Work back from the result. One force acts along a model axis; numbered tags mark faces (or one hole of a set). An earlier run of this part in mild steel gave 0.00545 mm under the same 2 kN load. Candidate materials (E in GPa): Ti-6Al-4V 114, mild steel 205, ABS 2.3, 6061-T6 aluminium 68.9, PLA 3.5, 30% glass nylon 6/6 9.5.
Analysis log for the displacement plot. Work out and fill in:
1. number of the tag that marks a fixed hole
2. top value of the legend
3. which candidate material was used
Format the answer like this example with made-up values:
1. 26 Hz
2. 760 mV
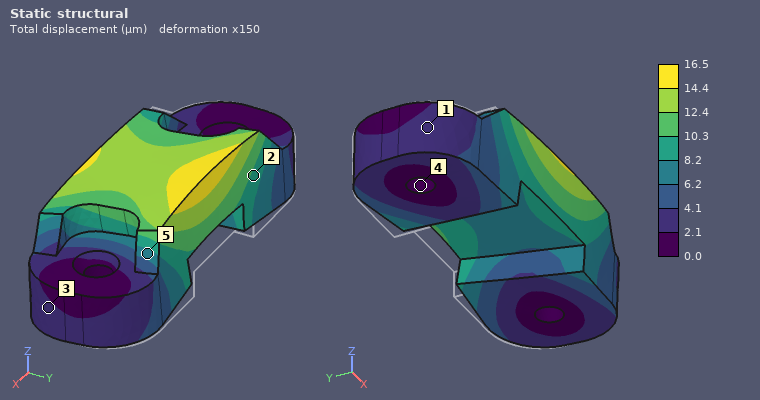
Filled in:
1. 4
2. 16.5 µm
3. 6061-T6 aluminium
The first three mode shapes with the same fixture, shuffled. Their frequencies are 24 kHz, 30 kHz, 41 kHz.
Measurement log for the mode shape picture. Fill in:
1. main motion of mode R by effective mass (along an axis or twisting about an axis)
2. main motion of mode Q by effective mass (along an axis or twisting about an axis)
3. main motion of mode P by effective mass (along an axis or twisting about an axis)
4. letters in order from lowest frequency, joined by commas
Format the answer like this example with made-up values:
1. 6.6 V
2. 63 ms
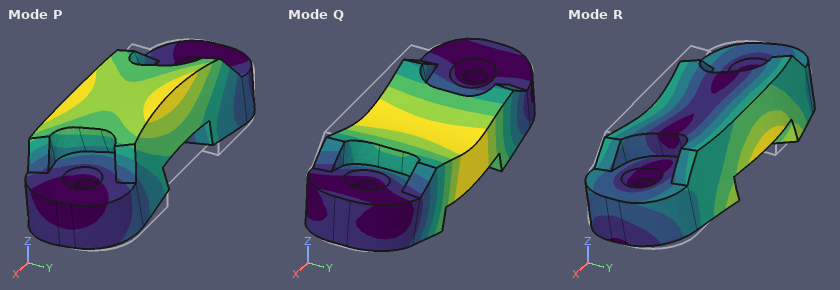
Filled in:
1. along Y
2. along Z
3. along Y
4. P, Q, R
